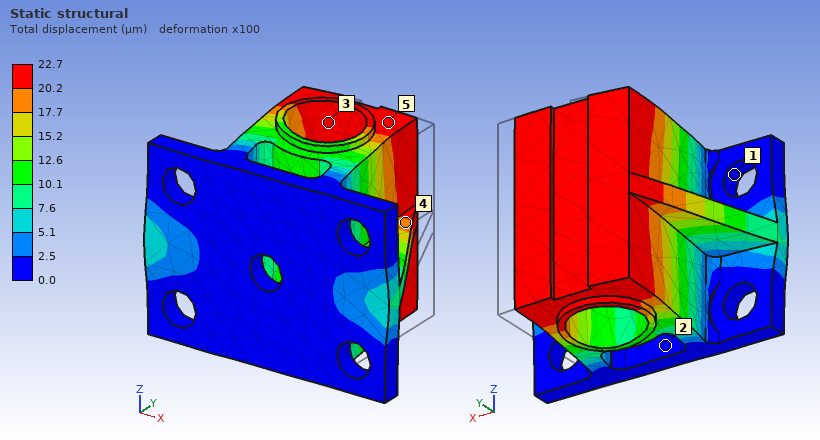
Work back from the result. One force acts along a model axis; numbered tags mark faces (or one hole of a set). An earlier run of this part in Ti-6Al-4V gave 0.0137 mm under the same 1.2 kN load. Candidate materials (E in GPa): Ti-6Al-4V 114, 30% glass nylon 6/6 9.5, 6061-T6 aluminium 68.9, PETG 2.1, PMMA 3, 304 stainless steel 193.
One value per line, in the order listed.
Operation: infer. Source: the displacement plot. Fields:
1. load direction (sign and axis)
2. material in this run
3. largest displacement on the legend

-X
6061-T6 aluminium
22.7 µm
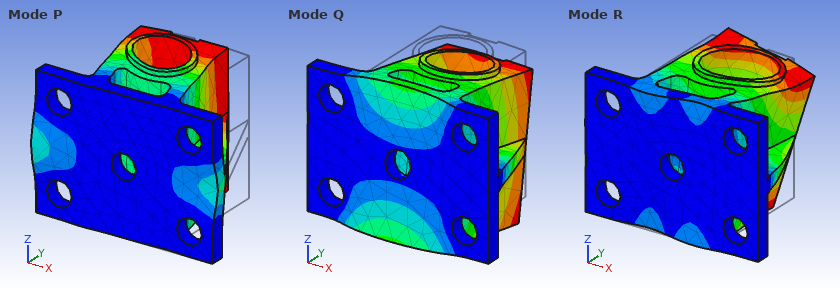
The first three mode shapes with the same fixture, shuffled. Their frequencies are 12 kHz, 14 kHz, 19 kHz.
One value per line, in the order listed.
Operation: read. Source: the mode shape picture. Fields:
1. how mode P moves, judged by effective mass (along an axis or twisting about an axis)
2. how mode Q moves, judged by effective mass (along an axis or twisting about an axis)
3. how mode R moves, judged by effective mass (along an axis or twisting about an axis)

along X
along Z
twisting about Y
